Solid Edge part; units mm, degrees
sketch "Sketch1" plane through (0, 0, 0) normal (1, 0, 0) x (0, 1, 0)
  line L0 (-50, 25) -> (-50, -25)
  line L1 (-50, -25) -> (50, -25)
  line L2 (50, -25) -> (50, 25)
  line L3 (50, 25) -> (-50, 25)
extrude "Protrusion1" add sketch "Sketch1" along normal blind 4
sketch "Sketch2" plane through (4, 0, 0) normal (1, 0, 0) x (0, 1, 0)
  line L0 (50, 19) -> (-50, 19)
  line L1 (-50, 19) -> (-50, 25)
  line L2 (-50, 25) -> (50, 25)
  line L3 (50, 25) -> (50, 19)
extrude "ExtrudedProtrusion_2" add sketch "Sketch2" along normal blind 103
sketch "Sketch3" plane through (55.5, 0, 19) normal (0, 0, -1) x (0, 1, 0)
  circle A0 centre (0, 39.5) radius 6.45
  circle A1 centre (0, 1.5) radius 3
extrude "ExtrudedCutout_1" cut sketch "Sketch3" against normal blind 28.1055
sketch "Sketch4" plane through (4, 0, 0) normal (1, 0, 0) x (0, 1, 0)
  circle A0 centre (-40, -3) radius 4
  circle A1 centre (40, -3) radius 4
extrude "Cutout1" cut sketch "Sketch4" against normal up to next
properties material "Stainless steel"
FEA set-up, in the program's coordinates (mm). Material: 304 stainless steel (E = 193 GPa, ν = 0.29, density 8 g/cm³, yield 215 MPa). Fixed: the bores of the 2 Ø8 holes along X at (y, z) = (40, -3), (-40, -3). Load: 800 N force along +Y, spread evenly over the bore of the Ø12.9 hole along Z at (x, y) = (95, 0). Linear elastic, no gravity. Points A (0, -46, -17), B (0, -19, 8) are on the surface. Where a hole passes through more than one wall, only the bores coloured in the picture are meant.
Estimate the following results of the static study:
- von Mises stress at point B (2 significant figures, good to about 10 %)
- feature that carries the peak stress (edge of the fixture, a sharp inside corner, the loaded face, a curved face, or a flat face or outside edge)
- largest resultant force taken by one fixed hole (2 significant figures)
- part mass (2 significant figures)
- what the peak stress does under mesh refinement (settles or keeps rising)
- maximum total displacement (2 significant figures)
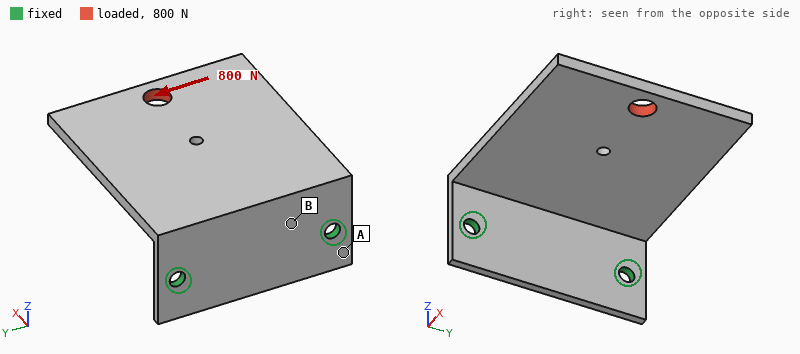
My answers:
32 MPa
edge of the fixture
1.0 kN
640 g
keeps rising
0.17 mm
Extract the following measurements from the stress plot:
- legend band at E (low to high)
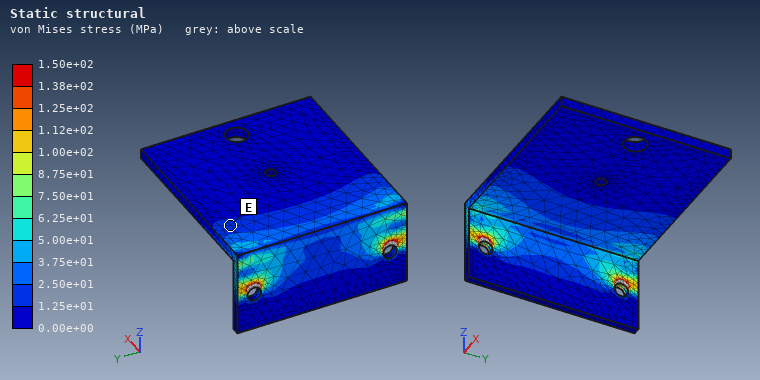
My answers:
1.25e+01 to 2.50e+01 MPa
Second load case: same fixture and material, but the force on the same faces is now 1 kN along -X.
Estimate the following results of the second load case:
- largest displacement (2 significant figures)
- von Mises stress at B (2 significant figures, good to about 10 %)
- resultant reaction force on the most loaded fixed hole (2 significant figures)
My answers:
0.35 mm
34 MPa
500 N
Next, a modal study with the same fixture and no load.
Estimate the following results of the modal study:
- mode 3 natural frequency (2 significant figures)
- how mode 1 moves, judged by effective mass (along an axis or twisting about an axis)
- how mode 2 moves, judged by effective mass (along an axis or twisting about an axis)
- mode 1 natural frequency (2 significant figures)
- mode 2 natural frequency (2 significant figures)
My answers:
1100 Hz
along Z
along Y
210 Hz
730 Hz
